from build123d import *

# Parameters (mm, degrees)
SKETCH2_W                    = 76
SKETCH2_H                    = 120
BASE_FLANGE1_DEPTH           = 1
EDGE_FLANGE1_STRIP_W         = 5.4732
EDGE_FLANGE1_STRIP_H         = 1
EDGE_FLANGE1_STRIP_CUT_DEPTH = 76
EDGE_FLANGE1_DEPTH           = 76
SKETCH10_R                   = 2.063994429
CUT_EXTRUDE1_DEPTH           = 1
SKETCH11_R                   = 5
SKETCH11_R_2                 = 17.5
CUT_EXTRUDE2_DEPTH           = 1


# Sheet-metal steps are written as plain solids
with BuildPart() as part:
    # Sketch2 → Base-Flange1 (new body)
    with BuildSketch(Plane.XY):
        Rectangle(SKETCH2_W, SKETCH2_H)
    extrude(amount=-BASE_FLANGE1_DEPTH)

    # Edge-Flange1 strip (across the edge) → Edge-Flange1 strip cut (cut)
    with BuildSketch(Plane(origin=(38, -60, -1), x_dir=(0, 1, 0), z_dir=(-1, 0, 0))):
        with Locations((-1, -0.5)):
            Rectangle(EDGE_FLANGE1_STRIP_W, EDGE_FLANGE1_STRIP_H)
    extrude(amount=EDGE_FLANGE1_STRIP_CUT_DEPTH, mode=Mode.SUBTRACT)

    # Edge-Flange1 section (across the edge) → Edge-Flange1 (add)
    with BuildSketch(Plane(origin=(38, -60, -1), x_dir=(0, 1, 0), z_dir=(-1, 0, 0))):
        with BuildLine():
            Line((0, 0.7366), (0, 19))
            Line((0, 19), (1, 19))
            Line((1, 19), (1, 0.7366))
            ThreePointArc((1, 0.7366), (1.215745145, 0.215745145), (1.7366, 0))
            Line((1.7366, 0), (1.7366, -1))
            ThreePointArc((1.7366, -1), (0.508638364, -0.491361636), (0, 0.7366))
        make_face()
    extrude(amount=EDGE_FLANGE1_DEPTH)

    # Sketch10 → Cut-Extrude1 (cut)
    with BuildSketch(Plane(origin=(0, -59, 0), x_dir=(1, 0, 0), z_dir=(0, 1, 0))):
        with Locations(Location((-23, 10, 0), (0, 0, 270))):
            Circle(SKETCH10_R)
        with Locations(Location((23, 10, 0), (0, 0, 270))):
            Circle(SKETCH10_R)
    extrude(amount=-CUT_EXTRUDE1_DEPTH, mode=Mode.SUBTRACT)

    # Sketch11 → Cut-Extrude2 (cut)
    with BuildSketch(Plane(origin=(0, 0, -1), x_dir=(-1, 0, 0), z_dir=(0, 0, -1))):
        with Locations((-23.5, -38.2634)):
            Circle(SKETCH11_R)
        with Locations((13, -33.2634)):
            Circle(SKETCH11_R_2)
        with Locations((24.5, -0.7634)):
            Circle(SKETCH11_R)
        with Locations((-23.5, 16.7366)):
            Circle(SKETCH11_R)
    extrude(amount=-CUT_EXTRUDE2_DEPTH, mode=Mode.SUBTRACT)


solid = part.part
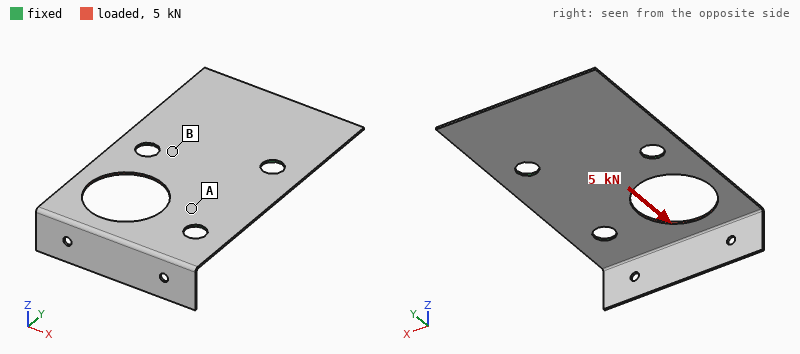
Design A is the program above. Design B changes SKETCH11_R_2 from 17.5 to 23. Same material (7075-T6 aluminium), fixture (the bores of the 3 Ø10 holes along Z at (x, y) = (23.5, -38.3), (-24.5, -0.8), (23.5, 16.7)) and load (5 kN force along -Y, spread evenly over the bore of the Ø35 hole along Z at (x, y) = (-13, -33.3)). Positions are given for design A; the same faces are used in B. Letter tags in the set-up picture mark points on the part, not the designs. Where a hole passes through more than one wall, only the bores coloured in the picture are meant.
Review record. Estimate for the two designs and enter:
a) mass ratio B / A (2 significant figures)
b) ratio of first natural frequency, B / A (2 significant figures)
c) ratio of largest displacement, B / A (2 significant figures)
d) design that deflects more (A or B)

0.92
0.95
3.8
B
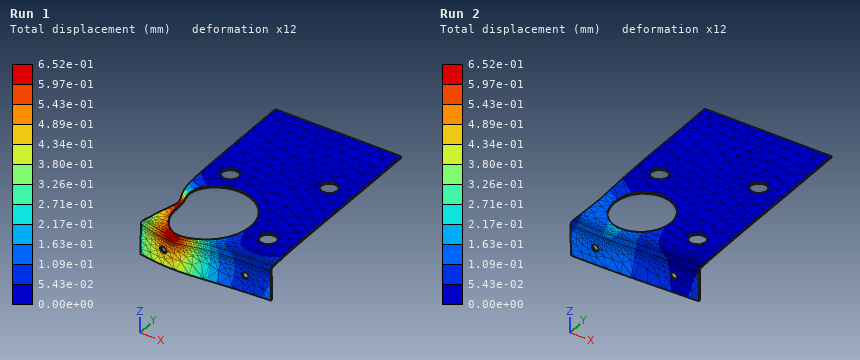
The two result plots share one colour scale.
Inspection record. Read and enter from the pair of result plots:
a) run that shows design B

Run 1
